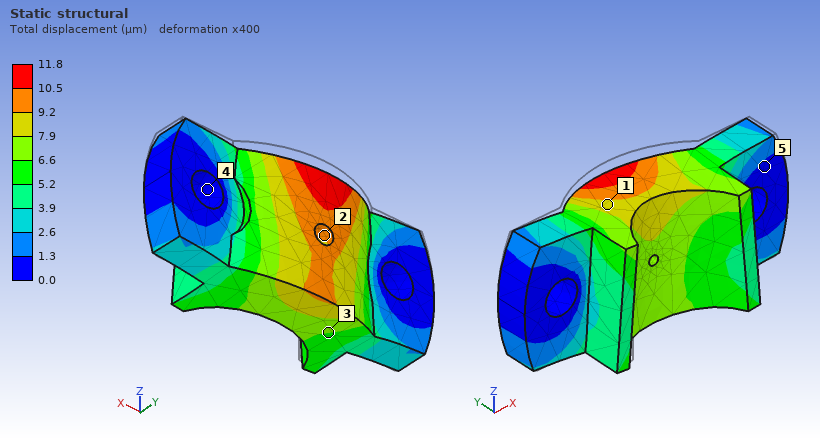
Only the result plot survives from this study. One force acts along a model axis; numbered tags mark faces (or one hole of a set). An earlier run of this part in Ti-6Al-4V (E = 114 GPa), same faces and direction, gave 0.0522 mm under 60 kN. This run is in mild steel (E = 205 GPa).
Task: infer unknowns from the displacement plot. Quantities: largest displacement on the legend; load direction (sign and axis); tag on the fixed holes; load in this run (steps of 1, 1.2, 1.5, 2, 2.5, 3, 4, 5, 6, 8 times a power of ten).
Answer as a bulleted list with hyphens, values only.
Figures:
- 11.8 µm
- -Z
- 4
- 25 kN
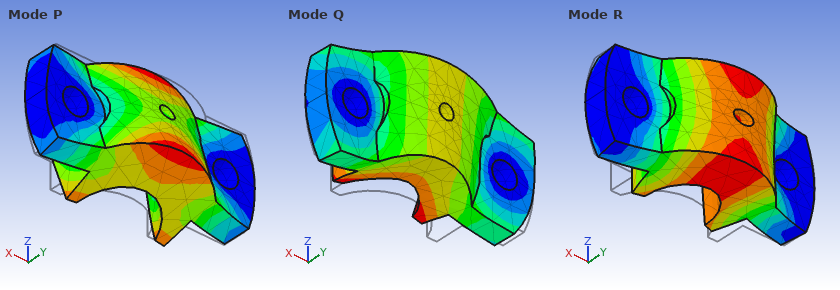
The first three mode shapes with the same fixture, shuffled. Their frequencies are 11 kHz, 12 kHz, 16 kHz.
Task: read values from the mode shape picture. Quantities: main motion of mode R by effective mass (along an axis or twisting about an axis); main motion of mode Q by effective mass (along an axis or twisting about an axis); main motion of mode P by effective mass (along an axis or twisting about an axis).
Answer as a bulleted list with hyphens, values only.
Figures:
- along Y
- along Z
- twisting about X
